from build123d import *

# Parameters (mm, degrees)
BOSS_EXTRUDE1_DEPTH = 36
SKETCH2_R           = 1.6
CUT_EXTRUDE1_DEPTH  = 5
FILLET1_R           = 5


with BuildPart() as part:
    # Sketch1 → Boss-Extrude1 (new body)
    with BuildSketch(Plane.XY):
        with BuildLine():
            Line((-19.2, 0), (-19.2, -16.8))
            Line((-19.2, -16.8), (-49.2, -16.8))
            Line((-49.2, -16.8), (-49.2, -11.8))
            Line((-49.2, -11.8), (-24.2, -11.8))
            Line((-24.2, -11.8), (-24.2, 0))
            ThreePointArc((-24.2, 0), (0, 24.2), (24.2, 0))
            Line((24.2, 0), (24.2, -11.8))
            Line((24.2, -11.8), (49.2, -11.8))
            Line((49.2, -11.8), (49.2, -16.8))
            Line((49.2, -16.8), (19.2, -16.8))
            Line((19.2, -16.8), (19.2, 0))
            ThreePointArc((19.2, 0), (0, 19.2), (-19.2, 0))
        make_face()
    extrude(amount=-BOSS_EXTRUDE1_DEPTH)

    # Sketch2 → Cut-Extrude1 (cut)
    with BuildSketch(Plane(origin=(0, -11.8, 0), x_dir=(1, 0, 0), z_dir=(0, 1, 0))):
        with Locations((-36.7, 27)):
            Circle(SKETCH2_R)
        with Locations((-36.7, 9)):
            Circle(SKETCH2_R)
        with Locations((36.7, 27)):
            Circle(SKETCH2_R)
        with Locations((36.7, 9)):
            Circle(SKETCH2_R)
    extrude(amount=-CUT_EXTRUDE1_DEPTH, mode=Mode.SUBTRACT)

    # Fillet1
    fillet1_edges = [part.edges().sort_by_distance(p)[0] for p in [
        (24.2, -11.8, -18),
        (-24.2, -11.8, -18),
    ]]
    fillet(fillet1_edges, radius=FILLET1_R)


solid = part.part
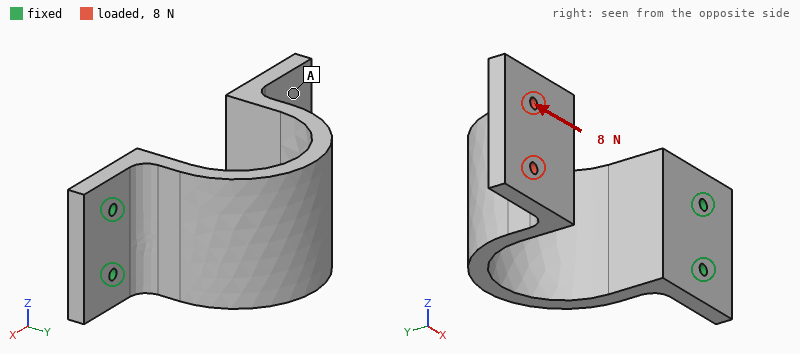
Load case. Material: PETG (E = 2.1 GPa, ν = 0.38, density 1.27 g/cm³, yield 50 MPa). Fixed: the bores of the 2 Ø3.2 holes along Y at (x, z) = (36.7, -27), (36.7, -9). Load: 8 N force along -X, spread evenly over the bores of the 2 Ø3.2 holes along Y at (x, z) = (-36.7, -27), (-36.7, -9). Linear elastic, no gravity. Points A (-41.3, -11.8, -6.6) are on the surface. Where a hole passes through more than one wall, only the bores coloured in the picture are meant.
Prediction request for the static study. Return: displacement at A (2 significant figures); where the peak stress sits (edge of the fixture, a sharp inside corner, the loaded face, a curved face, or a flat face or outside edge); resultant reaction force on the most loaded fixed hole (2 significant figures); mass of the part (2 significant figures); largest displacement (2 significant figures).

0.96 mm
a curved face
4.0 N
35 g
1.1 mm
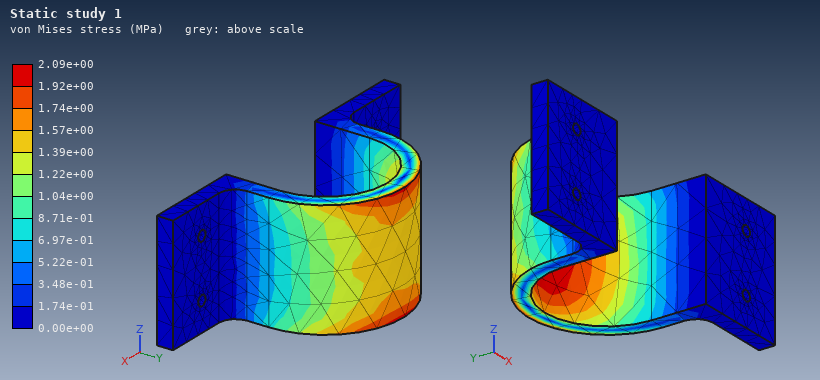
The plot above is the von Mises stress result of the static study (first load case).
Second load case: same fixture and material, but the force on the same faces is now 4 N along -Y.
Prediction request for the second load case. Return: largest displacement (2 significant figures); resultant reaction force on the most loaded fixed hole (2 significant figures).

1.3 mm
2.6 N
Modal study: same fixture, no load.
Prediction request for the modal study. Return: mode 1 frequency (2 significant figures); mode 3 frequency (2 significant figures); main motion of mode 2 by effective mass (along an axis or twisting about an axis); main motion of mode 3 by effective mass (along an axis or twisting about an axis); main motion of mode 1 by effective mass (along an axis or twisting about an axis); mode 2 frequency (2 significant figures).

92 Hz
220 Hz
along Z
along X
along Y
140 Hz
